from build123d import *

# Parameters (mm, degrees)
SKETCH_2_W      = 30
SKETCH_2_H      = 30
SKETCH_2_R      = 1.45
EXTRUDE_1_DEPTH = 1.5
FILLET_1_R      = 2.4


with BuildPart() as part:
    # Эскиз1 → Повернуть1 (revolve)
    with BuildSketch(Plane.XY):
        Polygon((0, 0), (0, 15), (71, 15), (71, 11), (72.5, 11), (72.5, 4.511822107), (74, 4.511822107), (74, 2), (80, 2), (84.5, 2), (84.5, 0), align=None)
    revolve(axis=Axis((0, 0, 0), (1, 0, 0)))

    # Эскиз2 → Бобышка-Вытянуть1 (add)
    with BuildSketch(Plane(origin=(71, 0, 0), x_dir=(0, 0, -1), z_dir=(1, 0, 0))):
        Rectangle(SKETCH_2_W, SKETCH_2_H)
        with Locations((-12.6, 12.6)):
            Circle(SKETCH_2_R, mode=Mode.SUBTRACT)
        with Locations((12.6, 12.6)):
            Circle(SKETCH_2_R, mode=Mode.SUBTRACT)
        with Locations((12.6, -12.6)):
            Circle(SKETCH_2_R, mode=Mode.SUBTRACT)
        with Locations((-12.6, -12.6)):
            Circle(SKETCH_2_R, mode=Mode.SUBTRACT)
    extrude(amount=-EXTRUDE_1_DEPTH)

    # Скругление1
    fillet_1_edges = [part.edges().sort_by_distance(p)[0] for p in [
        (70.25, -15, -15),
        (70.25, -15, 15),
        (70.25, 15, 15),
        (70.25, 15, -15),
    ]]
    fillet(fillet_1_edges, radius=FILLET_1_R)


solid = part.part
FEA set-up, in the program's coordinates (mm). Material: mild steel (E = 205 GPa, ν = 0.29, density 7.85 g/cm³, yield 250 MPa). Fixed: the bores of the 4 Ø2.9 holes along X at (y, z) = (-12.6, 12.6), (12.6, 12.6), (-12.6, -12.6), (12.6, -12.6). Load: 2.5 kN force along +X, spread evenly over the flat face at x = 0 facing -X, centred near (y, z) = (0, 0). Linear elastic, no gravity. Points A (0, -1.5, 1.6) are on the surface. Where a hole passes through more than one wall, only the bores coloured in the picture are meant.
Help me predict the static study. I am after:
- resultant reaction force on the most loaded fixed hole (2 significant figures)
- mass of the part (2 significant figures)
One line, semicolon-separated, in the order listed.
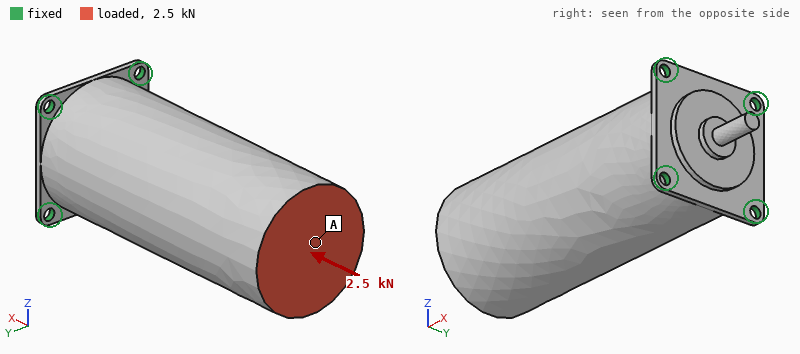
690 N; 400 g
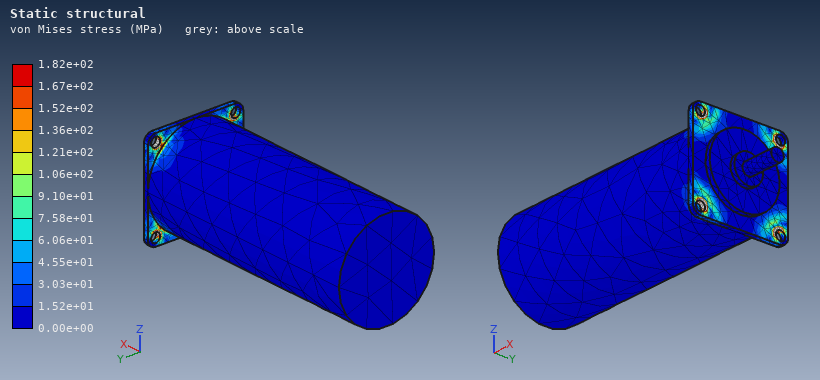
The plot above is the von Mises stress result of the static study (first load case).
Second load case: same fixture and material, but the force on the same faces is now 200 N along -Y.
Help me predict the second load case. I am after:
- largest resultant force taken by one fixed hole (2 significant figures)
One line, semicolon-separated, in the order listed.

330 N
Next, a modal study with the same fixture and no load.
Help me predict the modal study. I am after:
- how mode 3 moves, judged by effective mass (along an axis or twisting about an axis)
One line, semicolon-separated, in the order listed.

along X
